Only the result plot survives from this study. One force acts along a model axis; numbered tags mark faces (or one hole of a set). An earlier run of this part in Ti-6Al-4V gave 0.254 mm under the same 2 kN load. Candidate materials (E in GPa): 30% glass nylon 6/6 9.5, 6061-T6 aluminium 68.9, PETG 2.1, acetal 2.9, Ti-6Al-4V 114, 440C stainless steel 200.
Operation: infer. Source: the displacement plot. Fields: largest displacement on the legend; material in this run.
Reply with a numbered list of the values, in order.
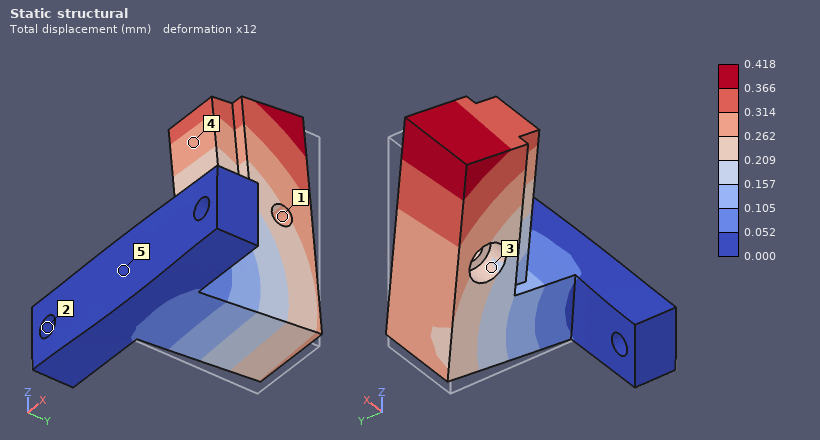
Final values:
1. 0.418 mm
2. 6061-T6 aluminium
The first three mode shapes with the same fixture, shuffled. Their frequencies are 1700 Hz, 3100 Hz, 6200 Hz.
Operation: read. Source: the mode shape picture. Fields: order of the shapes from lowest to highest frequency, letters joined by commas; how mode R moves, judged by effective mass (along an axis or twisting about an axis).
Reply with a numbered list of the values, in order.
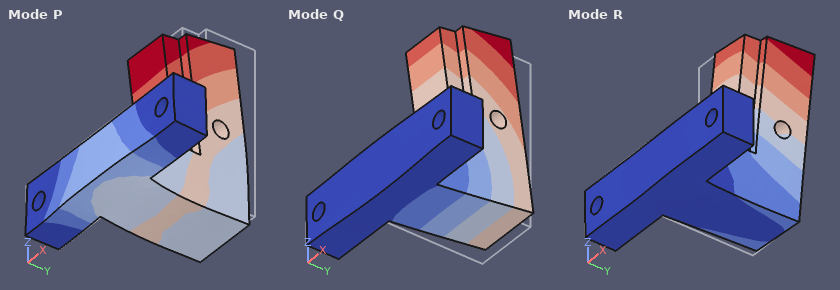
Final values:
1. Q, R, P
2. along X
